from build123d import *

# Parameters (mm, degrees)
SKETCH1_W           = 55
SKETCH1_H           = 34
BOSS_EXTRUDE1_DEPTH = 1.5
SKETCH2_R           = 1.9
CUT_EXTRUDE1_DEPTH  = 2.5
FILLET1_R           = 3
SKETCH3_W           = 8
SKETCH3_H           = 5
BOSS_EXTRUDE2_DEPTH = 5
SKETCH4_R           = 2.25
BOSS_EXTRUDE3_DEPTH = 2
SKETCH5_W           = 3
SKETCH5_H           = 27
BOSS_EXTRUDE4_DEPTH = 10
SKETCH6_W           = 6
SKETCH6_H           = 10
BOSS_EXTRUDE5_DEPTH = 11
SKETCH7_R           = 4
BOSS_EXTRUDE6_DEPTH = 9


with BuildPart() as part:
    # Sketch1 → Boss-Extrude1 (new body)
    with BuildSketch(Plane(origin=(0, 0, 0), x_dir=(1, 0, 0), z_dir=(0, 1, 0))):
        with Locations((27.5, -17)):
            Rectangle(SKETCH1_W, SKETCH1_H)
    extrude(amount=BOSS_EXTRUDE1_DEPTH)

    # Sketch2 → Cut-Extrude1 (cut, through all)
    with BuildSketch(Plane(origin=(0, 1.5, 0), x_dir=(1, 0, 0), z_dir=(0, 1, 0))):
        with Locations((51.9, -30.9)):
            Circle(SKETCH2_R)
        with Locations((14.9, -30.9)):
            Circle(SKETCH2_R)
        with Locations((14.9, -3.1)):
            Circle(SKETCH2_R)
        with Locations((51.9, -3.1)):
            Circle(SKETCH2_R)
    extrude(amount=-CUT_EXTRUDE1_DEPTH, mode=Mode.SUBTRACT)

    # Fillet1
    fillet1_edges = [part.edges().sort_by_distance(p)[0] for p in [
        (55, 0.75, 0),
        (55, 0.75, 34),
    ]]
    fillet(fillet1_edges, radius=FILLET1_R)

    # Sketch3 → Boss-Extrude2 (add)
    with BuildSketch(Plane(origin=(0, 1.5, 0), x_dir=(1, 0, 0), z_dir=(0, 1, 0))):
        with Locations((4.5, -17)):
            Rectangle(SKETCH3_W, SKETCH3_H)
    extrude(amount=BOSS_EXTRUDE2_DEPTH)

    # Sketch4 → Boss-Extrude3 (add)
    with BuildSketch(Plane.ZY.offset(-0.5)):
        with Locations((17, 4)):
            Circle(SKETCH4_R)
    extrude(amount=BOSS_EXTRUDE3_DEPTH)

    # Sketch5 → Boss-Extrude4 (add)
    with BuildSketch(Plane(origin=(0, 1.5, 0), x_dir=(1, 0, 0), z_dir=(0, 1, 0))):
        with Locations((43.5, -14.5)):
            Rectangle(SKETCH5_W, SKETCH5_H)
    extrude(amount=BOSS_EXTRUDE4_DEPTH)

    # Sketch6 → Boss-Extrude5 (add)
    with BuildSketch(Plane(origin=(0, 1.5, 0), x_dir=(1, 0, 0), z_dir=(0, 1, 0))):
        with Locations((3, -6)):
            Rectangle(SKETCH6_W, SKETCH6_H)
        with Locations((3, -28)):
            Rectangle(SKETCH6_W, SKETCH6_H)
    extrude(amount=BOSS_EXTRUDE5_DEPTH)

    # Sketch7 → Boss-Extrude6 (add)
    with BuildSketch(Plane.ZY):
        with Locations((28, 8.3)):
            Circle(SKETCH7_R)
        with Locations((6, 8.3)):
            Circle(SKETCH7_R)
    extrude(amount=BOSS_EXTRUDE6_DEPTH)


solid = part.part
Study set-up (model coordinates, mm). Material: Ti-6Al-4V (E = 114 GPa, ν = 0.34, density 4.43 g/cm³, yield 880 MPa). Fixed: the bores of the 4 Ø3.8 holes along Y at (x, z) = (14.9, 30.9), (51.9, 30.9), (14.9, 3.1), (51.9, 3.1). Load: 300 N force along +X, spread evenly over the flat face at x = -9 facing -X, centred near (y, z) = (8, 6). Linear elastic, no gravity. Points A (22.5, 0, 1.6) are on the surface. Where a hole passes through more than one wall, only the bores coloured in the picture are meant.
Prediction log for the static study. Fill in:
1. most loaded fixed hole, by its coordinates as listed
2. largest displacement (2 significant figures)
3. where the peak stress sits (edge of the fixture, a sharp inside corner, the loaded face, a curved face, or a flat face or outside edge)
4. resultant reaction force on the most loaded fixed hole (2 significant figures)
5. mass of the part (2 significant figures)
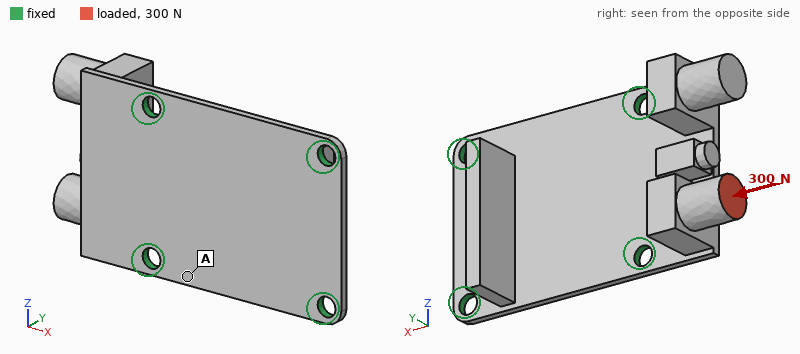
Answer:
(14.9, 3.1)
0.52 mm
a flat face or outside edge
240 N
27 g
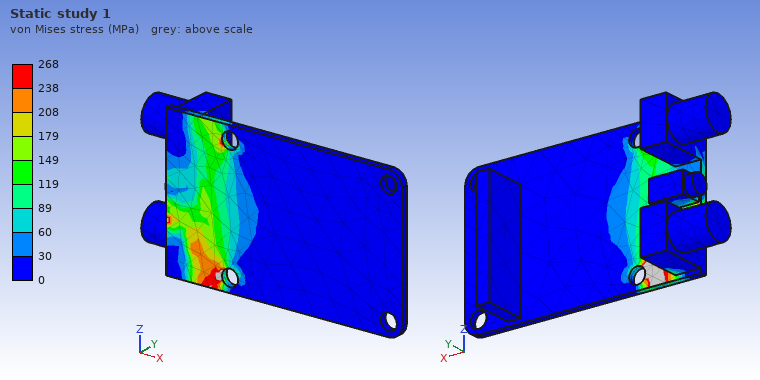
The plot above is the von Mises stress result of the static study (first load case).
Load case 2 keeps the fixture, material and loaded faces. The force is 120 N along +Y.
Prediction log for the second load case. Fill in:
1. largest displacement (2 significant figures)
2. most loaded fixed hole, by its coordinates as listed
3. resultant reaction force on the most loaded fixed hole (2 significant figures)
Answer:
0.54 mm
(14.9, 3.1)
110 N
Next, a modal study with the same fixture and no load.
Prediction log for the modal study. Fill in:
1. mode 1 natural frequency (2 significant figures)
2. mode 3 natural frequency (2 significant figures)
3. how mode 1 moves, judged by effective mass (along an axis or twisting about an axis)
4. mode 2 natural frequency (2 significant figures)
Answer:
1300 Hz
3700 Hz
along Y
2500 Hz
